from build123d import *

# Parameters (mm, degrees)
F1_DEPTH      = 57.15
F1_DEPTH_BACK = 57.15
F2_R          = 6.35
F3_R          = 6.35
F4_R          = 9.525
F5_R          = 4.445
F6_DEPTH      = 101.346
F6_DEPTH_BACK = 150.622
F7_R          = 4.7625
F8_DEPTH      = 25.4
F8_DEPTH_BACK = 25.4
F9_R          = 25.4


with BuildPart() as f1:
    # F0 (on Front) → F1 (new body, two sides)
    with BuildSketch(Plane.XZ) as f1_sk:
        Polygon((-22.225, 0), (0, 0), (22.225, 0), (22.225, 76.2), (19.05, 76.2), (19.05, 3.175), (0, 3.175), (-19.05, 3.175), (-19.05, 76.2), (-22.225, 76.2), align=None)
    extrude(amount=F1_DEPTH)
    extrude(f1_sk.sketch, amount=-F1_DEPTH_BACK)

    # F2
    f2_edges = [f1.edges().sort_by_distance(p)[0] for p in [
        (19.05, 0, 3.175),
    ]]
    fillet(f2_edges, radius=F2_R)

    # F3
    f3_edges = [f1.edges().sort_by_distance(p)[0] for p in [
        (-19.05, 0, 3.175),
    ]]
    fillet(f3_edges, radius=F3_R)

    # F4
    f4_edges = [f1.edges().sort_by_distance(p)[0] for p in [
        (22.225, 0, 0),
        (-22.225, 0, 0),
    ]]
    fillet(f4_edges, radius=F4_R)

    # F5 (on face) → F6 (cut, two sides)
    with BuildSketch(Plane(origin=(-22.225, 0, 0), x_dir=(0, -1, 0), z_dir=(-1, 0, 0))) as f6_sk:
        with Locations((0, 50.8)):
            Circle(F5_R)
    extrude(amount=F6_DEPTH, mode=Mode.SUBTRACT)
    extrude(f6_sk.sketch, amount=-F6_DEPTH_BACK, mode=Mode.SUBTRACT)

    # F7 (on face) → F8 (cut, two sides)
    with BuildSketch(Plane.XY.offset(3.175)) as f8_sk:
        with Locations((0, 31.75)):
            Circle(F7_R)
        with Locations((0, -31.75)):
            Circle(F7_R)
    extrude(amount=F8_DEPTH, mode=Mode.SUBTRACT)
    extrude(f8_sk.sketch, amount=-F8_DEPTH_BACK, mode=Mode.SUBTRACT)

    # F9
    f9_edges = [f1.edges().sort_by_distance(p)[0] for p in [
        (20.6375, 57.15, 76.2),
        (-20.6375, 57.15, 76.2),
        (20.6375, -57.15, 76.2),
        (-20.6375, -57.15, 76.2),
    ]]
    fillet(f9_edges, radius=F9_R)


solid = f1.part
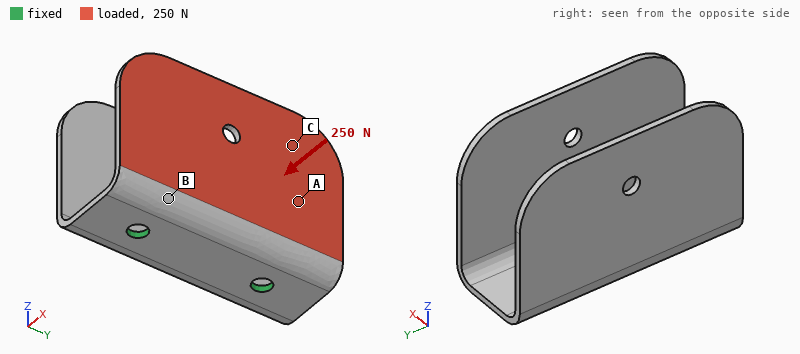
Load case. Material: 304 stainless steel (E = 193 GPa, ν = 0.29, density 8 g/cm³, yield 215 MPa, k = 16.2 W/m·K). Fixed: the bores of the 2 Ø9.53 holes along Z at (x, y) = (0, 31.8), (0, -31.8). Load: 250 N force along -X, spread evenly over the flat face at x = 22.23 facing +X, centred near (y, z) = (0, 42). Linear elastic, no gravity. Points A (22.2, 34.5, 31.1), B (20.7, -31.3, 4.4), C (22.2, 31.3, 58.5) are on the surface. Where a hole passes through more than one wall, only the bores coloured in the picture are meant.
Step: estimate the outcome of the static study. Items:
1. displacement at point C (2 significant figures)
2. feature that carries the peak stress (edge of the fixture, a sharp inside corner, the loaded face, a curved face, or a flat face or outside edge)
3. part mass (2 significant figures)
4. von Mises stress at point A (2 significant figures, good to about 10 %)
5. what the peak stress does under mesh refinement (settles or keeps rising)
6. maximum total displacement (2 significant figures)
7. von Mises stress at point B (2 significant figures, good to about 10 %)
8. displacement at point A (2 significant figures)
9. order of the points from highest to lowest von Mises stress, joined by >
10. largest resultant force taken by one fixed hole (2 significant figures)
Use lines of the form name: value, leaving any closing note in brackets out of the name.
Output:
displacement at point C: 0.30 mm
feature that carries the peak stress: edge of the fixture
part mass: 510 g
von Mises stress at point A: 17 MPa
what the peak stress does under mesh refinement: keeps rising
maximum total displacement: 0.42 mm
von Mises stress at point B: 36 MPa
displacement at point A: 0.14 mm
order of the points from highest to lowest von Mises stress, joined by >: B > A > C
largest resultant force taken by one fixed hole: 130 N
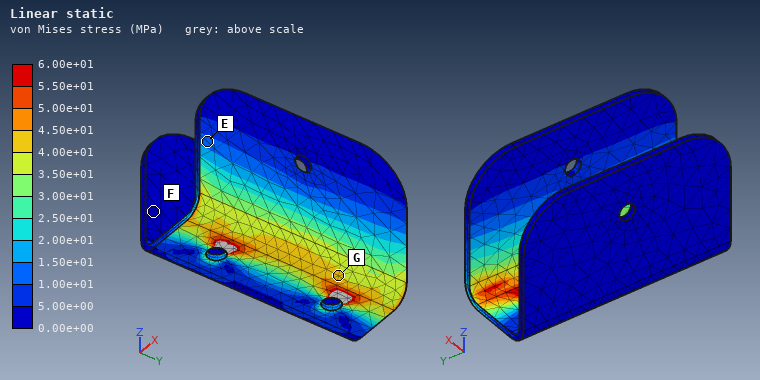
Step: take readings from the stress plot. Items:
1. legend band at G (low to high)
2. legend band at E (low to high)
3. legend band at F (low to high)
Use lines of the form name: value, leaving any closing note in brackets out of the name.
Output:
legend band at G: 4.00e+01 to 4.50e+01 MPa
legend band at E: 1.00e+01 to 1.50e+01 MPa
legend band at F: 0.00e+00 to 5.00e+00 MPa
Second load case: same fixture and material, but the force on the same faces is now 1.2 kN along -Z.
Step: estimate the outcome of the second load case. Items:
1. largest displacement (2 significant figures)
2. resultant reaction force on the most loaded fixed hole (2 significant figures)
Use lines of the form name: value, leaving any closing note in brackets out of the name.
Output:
largest displacement: 0.40 mm
resultant reaction force on the most loaded fixed hole: 600 N
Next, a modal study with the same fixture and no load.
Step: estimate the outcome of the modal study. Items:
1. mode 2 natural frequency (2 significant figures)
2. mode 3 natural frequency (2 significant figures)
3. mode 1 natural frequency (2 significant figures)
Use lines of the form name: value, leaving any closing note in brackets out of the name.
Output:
mode 2 natural frequency: 360 Hz
mode 3 natural frequency: 740 Hz
mode 1 natural frequency: 350 Hz
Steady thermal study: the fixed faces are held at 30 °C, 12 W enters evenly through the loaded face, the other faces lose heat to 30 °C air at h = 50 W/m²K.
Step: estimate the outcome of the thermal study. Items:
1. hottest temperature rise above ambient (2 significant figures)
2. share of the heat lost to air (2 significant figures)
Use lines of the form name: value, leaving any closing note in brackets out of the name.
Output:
hottest temperature rise above ambient: 25 K
share of the heat lost to air: 88 %
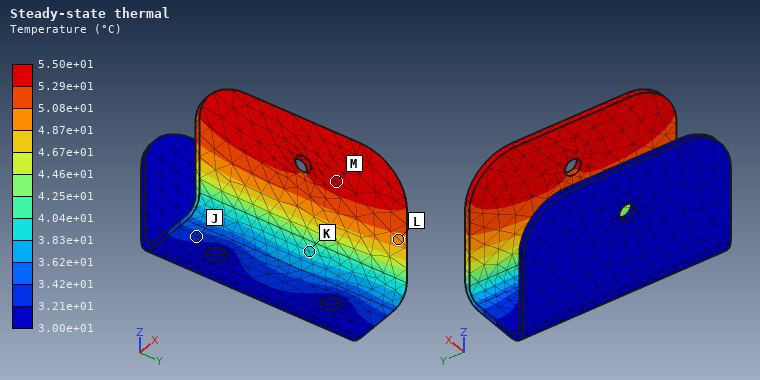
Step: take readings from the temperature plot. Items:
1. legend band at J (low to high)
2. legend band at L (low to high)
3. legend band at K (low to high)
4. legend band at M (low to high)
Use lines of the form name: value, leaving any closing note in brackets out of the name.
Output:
legend band at J: 3.21e+01 to 3.42e+01 °C
legend band at L: 4.87e+01 to 5.08e+01 °C
legend band at K: 3.83e+01 to 4.04e+01 °C
legend band at M: 5.29e+01 to 5.50e+01 °C
